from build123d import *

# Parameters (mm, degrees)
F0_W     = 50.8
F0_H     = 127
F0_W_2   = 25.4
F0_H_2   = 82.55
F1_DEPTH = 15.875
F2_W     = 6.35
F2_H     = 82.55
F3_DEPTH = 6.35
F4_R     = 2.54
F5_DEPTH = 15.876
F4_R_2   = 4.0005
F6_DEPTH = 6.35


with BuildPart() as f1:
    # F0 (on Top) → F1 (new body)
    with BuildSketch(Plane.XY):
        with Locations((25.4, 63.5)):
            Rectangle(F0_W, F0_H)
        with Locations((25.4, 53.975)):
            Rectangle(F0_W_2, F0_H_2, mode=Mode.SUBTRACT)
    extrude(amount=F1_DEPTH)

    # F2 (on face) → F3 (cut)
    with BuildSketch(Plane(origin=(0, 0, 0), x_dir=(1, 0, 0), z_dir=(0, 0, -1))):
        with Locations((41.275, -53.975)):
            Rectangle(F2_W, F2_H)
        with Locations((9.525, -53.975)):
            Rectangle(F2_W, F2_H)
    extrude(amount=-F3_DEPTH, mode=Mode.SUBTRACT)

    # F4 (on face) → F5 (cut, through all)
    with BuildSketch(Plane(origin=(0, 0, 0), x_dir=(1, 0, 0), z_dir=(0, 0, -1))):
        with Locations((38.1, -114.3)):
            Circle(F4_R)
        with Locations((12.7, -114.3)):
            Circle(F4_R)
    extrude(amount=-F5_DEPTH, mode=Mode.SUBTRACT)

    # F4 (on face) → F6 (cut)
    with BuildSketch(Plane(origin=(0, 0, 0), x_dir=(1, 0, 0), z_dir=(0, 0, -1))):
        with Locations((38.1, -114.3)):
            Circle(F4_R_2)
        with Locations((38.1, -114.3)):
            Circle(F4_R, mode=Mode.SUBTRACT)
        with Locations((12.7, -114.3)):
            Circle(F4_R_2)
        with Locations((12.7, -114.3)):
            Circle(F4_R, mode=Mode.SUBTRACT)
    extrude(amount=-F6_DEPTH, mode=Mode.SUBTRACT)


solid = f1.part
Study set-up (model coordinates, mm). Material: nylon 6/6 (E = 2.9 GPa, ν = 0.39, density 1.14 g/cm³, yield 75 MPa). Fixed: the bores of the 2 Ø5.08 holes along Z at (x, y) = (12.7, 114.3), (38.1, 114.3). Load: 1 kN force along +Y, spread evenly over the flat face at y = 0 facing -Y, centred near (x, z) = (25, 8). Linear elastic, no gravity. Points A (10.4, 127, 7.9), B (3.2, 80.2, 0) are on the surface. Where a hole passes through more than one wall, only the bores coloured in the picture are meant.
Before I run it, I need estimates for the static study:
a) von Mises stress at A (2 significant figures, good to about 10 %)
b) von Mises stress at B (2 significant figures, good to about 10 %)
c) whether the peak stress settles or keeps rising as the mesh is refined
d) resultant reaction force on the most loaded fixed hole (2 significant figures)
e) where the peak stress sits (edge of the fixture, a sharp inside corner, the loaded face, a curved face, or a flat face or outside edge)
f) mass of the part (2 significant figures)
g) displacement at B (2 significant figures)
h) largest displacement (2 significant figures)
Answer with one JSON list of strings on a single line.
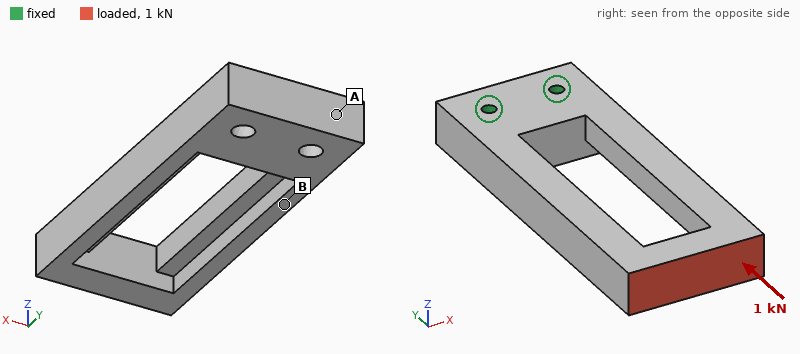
["1.1 MPa", "4.9 MPa", "keeps rising", "500 N", "edge of the fixture", "70 g", "0.10 mm", "0.62 mm"]
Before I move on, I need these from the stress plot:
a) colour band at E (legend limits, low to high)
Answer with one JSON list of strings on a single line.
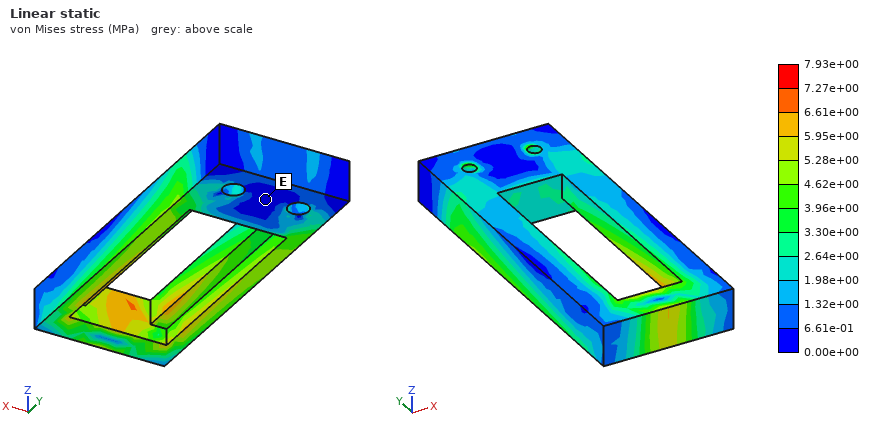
["0.00e+00 to 6.61e-01 MPa"]
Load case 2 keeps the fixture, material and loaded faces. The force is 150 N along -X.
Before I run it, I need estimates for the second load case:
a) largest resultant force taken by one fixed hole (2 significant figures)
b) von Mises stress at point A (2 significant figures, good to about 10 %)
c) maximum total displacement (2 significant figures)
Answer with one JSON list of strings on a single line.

["600 N", "1.3 MPa", "1.4 mm"]
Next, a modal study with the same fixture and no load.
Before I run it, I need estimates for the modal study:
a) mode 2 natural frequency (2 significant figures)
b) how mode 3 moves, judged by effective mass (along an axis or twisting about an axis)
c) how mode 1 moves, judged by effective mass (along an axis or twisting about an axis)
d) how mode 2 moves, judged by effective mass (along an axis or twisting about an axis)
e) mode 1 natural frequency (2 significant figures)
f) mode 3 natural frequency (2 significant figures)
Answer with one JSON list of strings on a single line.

["370 Hz", "twisting about Y", "along Z", "along X", "230 Hz", "640 Hz"]
